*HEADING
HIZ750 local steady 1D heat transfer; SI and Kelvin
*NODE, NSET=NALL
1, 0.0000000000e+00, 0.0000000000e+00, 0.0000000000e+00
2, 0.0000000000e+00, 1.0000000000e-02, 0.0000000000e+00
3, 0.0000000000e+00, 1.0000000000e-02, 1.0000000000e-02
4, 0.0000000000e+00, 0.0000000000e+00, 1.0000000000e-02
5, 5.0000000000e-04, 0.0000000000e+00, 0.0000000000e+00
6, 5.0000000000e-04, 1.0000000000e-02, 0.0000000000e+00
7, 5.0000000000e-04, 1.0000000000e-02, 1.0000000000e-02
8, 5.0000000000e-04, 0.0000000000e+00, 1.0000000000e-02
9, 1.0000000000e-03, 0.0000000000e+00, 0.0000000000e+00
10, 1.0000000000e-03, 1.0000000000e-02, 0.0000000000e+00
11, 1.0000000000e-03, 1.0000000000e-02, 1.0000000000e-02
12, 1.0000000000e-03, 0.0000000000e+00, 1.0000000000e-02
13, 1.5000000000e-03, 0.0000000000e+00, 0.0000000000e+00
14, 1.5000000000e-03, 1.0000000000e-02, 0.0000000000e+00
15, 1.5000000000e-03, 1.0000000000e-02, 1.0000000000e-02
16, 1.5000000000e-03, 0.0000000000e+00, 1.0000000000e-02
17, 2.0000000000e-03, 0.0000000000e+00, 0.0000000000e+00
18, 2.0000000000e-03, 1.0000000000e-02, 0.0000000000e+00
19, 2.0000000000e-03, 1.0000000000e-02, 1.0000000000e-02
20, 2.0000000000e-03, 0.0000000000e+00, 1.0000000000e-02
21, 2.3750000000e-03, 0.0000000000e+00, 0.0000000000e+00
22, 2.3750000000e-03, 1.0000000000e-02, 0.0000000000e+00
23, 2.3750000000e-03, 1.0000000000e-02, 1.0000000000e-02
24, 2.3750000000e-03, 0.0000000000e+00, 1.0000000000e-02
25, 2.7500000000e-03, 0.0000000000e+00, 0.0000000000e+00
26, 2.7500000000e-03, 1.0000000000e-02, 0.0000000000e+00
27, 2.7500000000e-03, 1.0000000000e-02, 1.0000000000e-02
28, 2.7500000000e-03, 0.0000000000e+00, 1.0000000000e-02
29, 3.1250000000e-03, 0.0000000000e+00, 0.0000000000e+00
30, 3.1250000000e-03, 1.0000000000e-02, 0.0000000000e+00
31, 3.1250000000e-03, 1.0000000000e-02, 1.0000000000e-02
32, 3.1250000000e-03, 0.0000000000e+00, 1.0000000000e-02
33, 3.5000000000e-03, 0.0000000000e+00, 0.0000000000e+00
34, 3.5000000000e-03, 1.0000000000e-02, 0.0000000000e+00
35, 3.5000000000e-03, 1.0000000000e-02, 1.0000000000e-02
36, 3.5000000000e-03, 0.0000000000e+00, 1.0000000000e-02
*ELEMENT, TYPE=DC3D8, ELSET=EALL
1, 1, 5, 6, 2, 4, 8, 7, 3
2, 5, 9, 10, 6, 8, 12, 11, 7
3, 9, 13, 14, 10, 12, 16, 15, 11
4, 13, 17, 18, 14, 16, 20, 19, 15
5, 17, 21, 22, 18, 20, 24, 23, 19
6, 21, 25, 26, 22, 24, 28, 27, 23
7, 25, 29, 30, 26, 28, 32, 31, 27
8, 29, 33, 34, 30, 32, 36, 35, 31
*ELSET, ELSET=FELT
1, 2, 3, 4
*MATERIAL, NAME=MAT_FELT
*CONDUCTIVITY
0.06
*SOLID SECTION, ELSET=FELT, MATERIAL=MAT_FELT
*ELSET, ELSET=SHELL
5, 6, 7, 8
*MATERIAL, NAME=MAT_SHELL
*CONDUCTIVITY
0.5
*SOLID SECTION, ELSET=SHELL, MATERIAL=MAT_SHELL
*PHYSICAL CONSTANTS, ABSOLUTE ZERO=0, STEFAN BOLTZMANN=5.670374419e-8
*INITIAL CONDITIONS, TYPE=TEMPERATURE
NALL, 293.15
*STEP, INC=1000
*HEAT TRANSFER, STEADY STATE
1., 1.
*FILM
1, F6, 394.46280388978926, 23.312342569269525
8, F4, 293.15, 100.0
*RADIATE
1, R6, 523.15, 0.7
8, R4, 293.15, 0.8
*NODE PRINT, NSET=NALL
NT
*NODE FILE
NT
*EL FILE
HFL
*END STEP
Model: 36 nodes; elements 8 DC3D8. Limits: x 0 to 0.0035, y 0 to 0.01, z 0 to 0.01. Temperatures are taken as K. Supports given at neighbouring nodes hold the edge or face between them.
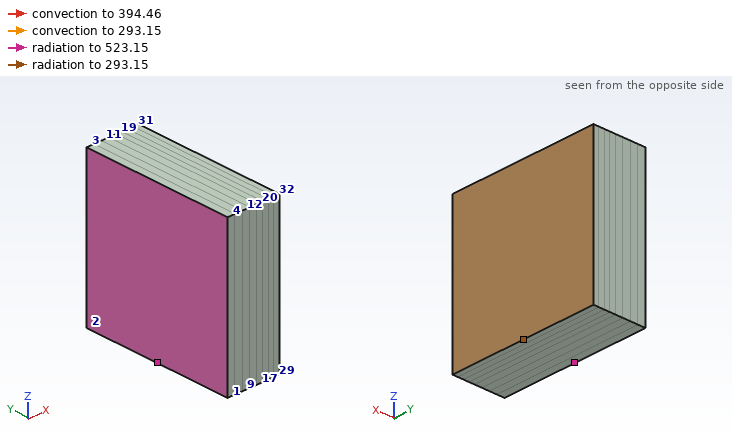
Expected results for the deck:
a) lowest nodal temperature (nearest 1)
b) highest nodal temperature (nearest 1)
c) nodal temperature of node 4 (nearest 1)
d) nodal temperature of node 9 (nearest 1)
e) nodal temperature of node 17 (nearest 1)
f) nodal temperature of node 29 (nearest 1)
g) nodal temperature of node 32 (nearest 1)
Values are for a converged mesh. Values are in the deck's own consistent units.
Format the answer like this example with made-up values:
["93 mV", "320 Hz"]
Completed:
["313 K", "391 K", "391 K", "355 K", "320 K", "315 K", "315 K"]
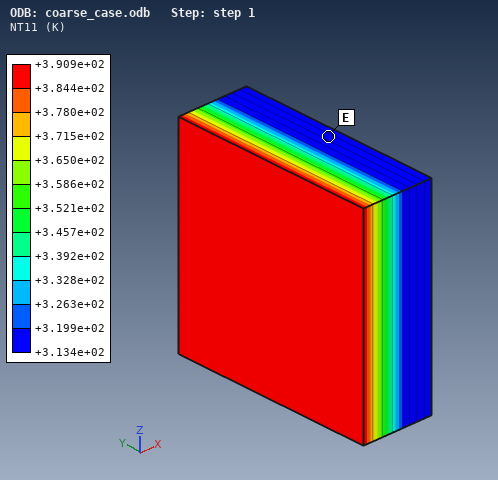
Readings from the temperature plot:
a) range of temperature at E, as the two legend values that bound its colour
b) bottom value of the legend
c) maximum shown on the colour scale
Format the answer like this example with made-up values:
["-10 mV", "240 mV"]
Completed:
["+3.134e+02 to +3.199e+02 K", "+3.134e+02 K", "+3.909e+02 K"]
